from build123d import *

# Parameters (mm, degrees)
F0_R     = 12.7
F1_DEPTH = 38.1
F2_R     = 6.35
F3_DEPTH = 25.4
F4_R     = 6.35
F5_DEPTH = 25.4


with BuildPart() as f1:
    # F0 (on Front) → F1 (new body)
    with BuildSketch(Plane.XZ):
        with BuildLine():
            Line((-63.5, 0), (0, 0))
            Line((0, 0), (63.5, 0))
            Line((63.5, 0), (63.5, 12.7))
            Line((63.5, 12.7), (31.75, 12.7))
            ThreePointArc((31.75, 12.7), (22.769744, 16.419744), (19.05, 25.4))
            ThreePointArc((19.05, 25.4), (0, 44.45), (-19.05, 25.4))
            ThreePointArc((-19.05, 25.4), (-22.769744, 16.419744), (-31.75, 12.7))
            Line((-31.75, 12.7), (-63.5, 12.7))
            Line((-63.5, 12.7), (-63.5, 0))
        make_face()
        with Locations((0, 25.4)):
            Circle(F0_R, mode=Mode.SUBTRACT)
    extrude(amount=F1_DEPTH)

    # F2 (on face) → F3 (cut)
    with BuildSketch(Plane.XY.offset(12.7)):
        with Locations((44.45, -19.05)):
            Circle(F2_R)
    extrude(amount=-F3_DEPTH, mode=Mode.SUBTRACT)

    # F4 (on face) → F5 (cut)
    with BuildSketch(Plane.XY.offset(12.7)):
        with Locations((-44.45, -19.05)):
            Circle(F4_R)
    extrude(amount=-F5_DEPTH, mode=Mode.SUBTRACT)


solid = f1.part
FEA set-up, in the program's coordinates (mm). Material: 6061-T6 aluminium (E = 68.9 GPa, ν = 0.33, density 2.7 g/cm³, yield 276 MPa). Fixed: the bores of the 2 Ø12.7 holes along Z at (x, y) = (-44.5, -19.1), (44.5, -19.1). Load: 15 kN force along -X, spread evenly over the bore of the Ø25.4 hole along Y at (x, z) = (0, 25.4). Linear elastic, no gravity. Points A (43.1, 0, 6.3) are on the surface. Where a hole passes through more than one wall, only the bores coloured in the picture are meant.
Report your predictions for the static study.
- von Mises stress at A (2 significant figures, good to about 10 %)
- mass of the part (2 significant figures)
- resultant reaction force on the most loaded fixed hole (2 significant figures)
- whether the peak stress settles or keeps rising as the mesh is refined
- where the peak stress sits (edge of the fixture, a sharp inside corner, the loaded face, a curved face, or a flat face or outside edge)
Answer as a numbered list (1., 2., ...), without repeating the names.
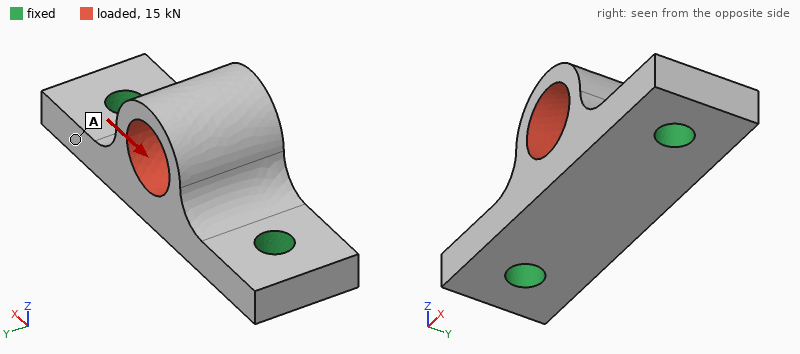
1. 9.5 MPa
2. 220 g
3. 8.5 kN
4. keeps rising
5. edge of the fixture
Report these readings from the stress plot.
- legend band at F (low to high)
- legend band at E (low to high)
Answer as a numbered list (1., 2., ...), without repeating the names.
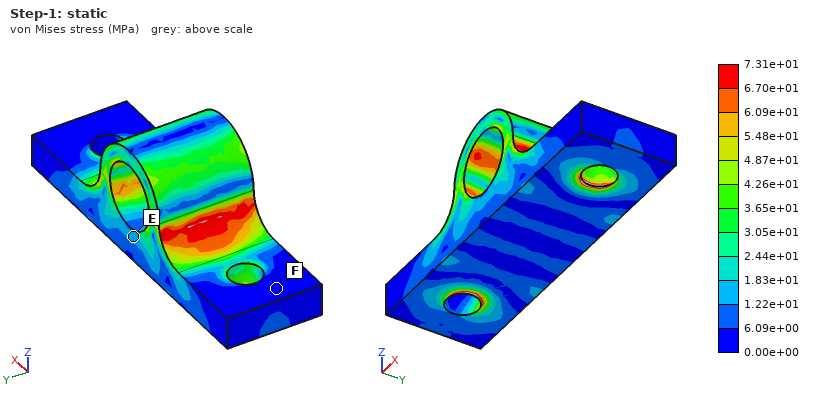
1. 0.00e+00 to 6.09e+00 MPa
2. 1.22e+01 to 1.83e+01 MPa
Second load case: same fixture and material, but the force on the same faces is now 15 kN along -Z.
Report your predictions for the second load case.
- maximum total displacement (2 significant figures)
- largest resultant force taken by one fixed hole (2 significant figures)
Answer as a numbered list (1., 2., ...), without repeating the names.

1. 65 µm
2. 8.0 kN
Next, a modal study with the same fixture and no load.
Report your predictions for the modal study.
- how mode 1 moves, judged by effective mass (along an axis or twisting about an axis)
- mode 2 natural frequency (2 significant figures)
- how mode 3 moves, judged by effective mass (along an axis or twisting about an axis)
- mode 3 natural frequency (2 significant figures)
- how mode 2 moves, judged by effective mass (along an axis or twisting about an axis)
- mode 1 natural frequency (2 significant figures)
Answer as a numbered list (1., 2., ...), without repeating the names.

1. along Y
2. 7400 Hz
3. along X
4. 10 kHz
5. along Z
6. 5300 Hz
